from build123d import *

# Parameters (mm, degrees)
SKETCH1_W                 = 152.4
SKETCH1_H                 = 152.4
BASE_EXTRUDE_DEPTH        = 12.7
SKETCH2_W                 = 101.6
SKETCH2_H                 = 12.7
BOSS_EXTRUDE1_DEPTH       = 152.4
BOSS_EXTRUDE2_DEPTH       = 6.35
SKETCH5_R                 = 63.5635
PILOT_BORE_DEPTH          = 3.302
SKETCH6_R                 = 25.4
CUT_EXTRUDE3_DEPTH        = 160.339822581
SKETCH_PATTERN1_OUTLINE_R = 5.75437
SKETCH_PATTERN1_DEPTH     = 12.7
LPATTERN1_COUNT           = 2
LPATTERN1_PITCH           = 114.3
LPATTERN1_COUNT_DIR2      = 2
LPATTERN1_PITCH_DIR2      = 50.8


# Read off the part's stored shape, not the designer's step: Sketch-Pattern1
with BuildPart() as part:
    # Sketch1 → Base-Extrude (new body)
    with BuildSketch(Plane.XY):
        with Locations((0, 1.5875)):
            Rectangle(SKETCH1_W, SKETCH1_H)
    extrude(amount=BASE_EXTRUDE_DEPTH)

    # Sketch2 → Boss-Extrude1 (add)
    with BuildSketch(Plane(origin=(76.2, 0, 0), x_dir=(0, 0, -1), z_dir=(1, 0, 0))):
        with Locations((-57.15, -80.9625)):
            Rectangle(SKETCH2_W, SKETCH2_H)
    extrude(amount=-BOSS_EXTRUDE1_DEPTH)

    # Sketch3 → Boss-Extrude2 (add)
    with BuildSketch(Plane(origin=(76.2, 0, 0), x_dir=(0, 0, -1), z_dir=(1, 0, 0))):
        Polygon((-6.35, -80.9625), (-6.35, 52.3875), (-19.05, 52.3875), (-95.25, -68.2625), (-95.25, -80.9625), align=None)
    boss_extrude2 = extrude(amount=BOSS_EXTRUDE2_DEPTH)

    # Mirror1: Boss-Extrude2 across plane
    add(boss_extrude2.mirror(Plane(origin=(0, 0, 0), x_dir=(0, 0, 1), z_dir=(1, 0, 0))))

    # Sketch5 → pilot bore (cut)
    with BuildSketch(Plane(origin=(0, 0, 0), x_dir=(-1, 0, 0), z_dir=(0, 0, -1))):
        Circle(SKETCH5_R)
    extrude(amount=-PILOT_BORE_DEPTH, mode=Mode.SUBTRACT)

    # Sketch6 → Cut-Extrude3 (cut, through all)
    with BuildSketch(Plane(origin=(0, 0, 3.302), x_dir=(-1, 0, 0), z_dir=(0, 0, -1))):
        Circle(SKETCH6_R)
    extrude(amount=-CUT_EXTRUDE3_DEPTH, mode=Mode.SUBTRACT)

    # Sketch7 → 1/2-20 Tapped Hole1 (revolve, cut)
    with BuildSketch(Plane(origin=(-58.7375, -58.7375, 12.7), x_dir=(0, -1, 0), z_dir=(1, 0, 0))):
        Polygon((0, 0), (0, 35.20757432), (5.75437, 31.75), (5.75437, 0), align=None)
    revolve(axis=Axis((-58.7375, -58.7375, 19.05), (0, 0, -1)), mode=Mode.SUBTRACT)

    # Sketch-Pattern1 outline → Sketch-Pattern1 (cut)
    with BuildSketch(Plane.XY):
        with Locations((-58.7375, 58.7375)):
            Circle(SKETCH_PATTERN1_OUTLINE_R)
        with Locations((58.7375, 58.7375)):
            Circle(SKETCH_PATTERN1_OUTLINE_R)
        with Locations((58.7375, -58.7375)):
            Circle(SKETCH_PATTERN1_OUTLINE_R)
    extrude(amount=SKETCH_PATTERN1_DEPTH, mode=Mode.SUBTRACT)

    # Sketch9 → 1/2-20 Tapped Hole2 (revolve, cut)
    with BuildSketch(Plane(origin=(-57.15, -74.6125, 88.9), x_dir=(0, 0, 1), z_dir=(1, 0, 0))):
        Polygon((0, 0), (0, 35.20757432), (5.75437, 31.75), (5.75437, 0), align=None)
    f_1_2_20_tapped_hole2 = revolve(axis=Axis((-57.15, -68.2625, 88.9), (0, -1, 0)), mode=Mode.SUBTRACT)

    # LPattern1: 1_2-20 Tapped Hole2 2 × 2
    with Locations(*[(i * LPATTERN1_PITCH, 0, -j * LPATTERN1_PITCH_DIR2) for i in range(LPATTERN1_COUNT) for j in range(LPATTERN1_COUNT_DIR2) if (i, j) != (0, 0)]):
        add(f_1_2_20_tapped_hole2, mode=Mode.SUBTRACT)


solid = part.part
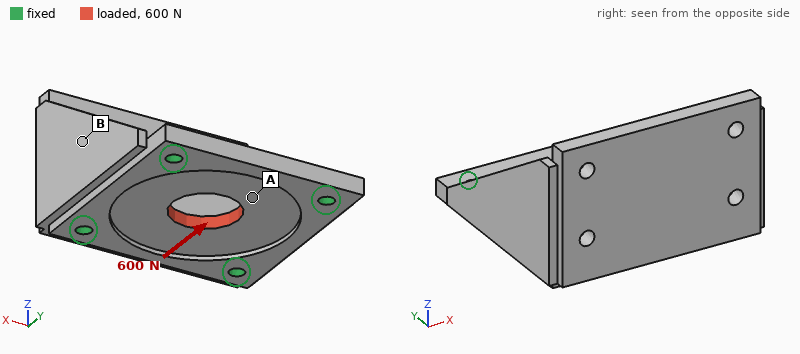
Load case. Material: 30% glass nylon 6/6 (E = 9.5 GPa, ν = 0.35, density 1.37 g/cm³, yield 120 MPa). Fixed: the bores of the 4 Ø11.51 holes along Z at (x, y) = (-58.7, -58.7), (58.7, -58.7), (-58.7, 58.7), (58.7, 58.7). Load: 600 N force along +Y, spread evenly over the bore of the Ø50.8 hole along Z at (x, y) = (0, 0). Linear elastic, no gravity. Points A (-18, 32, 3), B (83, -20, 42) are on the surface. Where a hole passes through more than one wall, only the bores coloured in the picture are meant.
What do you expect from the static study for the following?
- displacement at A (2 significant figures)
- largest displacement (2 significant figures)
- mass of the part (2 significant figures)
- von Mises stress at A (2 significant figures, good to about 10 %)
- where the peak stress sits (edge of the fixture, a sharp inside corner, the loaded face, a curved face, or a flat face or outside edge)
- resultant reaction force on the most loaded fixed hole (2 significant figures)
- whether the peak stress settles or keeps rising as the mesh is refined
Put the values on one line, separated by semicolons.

3.0 µm; 4.0 µm; 700 g; 0.37 MPa; edge of the fixture; 160 N; keeps rising
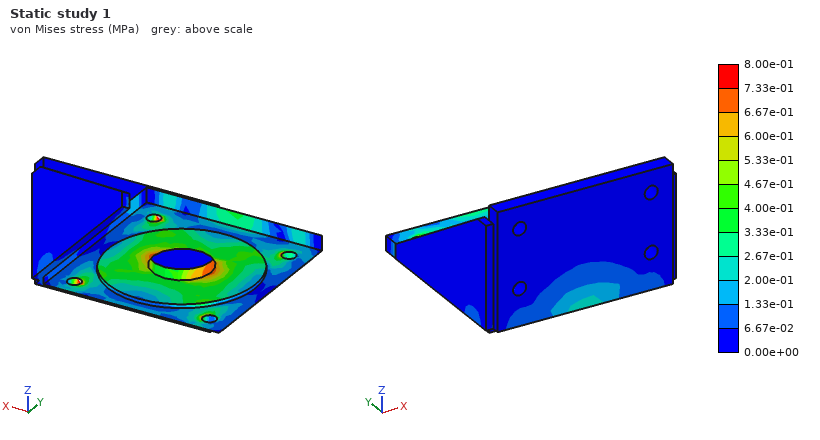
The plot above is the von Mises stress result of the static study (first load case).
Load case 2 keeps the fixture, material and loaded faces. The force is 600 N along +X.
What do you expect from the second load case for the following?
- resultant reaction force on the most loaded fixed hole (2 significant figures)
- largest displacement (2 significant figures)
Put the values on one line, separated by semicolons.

160 N; 3.8 µm
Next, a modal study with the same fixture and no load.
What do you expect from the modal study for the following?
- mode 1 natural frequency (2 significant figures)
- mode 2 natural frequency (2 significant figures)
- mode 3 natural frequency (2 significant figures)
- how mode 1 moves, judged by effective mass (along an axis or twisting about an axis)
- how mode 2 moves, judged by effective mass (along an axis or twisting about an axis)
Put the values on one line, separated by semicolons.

750 Hz; 1400 Hz; 1500 Hz; along Y; along X
